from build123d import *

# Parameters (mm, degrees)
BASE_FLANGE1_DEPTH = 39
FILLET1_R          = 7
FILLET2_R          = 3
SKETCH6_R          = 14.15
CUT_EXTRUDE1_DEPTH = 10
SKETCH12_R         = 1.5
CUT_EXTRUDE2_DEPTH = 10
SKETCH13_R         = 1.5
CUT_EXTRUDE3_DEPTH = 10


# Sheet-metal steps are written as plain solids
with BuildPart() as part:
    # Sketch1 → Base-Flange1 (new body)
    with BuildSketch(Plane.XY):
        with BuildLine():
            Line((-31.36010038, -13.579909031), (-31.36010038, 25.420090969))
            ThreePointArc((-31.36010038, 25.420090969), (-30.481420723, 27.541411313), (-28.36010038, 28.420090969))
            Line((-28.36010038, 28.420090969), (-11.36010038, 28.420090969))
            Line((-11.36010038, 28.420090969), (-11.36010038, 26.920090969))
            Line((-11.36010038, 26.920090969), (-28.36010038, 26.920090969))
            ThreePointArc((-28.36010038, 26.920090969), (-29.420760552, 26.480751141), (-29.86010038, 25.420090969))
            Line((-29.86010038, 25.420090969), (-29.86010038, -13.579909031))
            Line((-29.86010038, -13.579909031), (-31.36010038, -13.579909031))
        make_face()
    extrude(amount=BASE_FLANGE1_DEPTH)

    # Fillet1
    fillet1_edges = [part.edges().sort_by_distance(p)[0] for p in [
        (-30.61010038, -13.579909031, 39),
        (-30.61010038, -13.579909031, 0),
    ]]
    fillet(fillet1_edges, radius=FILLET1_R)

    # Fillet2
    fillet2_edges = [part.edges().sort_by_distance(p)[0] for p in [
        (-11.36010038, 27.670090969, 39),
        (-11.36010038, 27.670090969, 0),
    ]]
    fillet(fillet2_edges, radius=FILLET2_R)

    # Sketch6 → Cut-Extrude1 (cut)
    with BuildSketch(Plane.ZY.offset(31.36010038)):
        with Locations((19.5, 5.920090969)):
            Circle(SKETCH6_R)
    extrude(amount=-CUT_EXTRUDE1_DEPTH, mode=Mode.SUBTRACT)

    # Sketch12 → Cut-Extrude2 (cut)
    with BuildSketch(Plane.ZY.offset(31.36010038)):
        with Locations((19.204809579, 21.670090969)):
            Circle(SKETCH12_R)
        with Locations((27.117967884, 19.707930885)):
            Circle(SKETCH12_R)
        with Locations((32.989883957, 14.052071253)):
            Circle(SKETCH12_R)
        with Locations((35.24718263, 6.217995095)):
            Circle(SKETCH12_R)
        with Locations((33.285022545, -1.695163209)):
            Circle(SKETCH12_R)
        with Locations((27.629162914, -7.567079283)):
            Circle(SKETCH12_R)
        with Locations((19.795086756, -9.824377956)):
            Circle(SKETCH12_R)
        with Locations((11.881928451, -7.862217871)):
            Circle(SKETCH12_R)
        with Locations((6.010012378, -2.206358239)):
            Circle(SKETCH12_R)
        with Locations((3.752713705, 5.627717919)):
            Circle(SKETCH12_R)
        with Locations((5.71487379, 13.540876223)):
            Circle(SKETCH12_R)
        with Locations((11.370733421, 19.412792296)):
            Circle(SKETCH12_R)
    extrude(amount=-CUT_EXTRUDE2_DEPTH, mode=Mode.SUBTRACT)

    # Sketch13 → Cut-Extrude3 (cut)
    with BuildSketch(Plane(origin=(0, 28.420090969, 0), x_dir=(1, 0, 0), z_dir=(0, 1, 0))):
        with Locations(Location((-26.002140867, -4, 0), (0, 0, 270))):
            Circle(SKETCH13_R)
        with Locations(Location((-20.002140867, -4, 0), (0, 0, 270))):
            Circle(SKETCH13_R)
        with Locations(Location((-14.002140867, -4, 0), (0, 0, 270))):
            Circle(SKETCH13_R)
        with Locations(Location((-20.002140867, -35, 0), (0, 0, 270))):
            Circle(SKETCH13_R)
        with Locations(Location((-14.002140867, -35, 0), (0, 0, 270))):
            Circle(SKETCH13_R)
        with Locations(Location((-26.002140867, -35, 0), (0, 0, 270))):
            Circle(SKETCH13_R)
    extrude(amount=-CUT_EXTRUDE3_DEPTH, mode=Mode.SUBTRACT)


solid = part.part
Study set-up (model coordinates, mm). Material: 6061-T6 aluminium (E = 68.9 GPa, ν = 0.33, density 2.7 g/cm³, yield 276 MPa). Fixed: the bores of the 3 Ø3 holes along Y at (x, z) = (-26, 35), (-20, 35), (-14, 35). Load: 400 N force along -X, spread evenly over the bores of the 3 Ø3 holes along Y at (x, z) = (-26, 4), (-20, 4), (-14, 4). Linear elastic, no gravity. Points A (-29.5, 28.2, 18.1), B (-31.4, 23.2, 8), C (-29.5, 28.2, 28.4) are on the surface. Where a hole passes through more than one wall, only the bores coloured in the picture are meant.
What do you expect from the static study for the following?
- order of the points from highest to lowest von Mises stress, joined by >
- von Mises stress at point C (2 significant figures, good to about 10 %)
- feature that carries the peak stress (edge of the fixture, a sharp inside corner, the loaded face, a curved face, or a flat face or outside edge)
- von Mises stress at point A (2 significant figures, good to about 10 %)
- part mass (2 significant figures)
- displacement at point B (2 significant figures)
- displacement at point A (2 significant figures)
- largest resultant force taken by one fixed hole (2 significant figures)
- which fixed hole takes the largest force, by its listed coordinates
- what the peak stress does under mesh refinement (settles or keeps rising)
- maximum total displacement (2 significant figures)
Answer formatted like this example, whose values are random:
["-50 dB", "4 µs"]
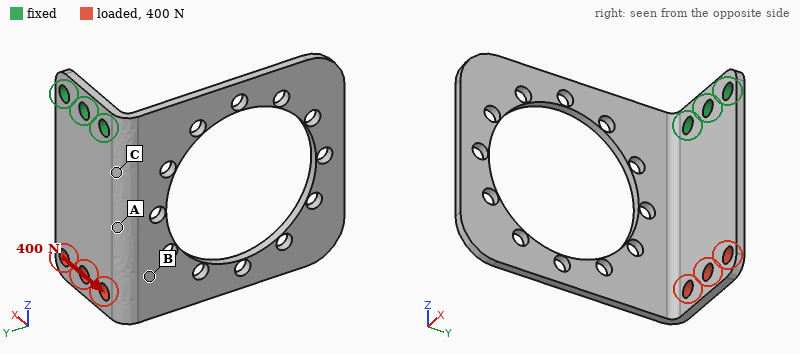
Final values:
["C > A > B", "68 MPa", "edge of the fixture", "44 MPa", "6.2 g", "0.081 mm", "0.044 mm", "940 N", "(-26, 35)", "keeps rising", "0.12 mm"]
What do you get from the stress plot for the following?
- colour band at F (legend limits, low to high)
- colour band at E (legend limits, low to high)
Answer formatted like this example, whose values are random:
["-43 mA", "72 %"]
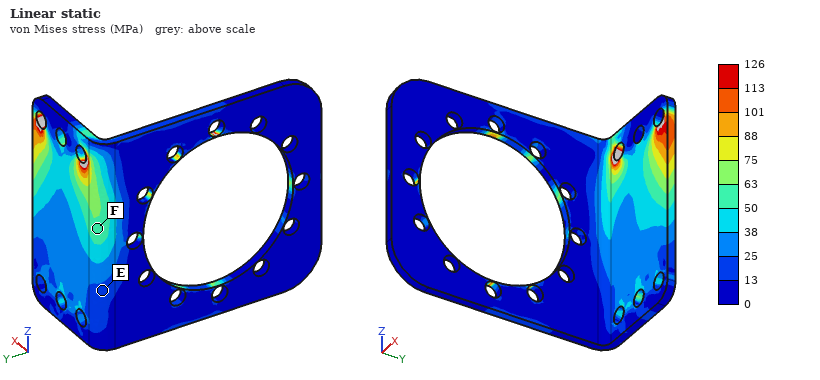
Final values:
["50 to 63 MPa", "13 to 25 MPa"]
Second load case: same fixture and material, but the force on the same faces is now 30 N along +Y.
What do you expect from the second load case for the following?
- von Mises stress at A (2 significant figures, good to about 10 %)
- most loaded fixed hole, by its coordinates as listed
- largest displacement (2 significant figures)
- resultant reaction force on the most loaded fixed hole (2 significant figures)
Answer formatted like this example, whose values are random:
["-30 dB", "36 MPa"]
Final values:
["17 MPa", "(-20, 35)", "0.29 mm", "24 N"]
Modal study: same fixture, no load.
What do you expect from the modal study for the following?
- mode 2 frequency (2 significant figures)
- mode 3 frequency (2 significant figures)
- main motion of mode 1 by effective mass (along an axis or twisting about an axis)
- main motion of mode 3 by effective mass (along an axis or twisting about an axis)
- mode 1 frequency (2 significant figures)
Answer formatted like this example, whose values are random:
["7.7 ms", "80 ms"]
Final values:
["930 Hz", "1300 Hz", "along X", "twisting about Y", "500 Hz"]
